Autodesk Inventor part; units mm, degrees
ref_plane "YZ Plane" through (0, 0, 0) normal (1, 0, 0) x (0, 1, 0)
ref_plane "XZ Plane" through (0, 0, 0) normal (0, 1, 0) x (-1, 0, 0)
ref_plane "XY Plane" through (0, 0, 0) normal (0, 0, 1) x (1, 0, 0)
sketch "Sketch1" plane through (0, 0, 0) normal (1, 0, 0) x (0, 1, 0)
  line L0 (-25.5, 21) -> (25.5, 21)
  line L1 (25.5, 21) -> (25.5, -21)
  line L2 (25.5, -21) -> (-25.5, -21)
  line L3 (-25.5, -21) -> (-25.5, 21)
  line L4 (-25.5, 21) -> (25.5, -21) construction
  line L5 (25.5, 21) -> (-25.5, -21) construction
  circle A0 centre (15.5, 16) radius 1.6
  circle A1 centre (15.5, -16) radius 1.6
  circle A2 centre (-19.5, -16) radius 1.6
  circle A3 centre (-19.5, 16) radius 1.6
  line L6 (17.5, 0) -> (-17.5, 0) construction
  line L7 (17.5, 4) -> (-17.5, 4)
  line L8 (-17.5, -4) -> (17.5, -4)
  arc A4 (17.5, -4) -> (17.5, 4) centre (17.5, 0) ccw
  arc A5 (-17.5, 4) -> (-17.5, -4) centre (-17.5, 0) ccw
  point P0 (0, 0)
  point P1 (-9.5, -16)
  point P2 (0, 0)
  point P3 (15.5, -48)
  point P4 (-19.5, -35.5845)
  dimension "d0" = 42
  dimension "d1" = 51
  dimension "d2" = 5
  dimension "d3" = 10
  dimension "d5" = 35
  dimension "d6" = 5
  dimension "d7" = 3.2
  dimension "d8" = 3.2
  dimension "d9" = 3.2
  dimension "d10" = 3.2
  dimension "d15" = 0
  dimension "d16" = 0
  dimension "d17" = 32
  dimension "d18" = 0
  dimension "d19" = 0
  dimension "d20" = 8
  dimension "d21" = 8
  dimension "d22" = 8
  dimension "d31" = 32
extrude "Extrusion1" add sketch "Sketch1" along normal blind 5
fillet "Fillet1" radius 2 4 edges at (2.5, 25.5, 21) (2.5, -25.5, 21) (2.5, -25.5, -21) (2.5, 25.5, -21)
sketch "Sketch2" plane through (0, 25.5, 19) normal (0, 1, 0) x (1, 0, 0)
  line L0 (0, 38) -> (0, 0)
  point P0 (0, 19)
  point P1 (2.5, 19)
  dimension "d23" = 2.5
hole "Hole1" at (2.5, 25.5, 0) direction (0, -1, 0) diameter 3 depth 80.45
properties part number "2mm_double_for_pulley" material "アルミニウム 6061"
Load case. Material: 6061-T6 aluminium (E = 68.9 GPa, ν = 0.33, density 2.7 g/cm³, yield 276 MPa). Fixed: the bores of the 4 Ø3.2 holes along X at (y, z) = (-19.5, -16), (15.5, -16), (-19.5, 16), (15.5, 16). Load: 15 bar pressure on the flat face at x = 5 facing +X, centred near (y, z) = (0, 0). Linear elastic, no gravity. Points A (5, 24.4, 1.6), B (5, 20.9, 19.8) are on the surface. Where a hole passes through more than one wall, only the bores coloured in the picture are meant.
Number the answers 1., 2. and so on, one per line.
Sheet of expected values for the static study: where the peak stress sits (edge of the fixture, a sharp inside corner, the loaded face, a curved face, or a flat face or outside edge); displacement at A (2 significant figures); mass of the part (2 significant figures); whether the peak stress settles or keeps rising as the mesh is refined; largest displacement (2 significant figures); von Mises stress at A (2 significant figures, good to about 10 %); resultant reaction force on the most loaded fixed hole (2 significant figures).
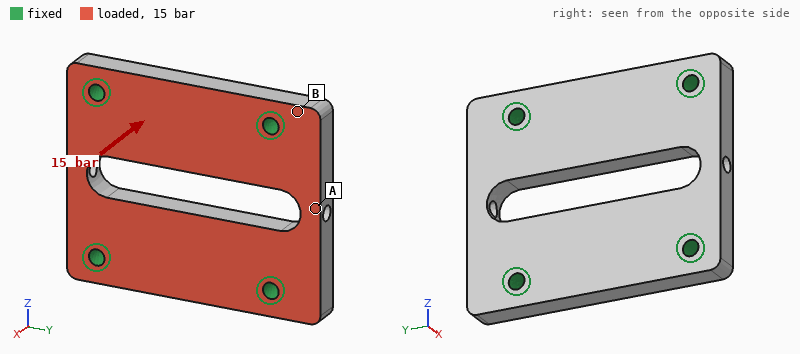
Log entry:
1. edge of the fixture
2. 9.9 µm
3. 24 g
4. keeps rising
5. 22 µm
6. 20 MPa
7. 720 N
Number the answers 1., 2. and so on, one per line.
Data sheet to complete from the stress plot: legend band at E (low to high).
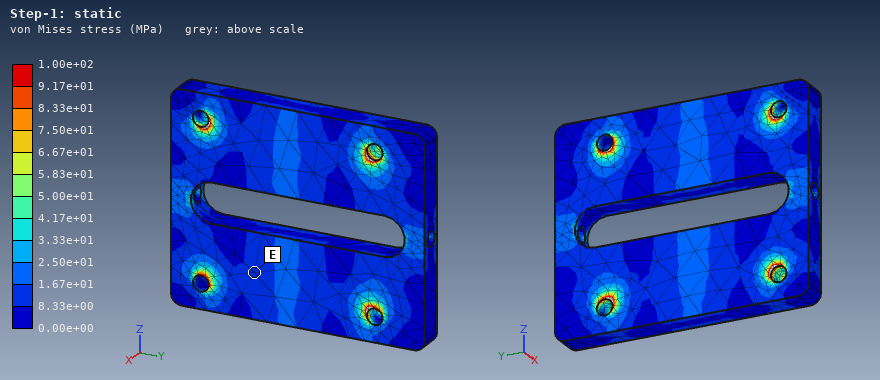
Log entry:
1. 8.33e+00 to 1.67e+01 MPa
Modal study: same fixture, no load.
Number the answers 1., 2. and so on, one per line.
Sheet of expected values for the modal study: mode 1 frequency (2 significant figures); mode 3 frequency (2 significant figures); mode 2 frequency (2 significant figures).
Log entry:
1. 15 kHz
2. 20 kHz
3. 15 kHz
